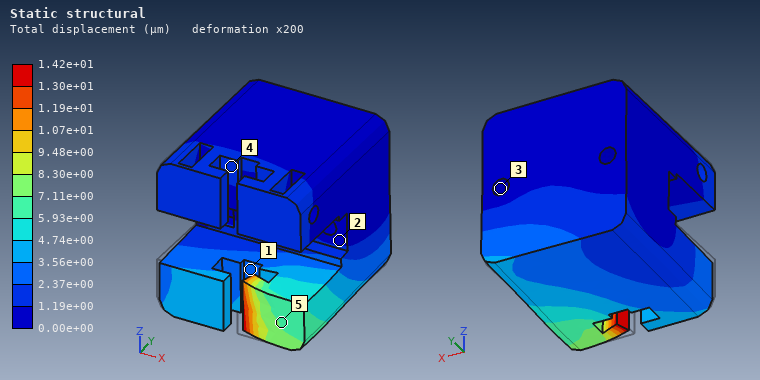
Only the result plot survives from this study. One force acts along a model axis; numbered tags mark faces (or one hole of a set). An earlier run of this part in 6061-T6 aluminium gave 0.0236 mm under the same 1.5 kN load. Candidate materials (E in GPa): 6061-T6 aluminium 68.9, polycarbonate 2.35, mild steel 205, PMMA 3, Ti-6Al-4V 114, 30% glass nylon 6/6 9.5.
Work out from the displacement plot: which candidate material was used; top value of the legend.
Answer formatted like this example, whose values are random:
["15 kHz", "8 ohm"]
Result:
["Ti-6Al-4V", "1.42e+01 µm"]
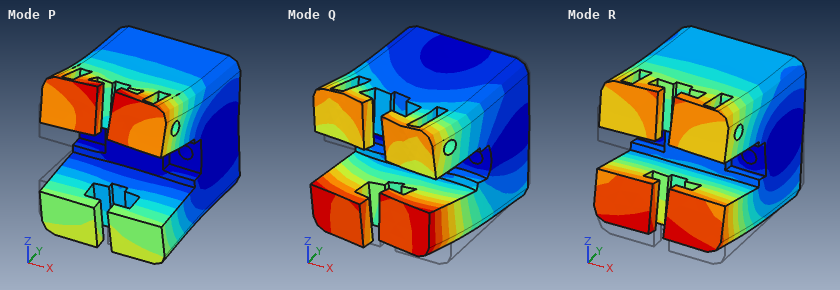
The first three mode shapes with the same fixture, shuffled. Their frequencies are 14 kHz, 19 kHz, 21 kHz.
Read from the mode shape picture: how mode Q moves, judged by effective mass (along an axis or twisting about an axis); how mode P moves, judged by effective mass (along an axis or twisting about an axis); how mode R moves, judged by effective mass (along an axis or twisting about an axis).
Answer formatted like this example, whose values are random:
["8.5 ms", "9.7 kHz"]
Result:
["along X", "along Y", "along Z"]
